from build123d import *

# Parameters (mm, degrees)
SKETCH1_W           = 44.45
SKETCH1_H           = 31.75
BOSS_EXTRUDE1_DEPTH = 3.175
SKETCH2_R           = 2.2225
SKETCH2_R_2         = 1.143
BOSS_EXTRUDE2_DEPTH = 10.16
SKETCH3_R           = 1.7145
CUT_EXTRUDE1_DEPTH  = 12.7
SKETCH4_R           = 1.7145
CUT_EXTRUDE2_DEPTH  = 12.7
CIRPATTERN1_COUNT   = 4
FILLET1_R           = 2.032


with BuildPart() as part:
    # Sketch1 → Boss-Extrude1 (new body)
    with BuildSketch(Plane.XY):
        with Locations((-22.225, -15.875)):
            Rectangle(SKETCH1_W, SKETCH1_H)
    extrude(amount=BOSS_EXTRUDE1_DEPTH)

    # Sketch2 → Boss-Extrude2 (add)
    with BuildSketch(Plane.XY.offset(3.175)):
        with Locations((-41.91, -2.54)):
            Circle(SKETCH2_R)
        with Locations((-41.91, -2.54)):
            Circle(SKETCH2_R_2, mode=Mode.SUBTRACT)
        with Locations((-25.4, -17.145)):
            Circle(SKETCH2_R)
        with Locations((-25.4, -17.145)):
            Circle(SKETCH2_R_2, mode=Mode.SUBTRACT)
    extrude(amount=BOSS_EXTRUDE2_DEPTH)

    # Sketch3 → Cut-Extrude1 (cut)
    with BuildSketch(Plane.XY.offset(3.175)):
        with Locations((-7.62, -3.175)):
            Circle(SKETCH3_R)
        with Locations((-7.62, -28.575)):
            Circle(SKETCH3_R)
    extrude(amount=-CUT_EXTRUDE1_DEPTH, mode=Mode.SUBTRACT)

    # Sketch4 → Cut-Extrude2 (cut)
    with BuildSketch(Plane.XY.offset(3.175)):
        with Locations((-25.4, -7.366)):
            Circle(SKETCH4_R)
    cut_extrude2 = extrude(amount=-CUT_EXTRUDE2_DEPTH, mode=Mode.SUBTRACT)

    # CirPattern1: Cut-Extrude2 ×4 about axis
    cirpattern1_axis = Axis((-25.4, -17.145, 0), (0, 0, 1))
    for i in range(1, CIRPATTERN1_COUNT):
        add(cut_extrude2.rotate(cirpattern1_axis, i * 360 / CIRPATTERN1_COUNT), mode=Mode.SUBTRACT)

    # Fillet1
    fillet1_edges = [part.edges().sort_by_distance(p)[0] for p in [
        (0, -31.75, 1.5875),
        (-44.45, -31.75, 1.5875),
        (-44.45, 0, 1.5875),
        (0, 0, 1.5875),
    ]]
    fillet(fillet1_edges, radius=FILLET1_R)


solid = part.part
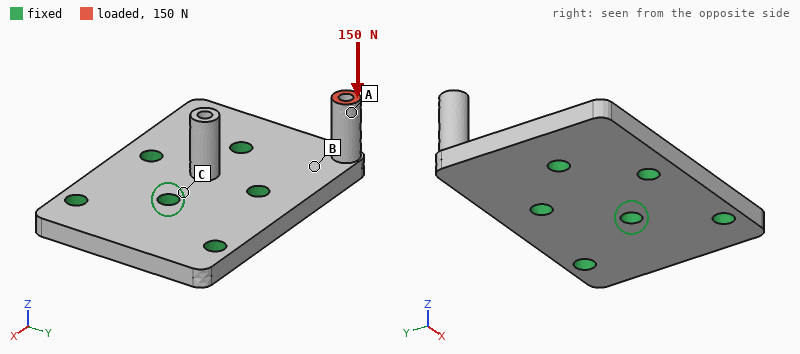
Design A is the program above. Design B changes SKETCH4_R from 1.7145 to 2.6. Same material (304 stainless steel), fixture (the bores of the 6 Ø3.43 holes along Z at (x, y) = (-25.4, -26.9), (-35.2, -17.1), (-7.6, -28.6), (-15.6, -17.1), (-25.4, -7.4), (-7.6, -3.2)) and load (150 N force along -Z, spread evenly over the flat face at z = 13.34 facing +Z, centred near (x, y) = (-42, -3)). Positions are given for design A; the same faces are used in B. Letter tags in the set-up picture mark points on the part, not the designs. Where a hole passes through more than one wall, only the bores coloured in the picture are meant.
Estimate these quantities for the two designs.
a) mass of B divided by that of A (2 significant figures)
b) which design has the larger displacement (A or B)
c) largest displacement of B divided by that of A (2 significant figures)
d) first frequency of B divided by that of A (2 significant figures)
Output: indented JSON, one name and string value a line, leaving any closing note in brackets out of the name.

{
  "mass of B divided by that of A": "0.97",
  "which design has the larger displacement": "A",
  "largest displacement of B divided by that of A": "0.88",
  "first frequency of B divided by that of A": "1.1"
}
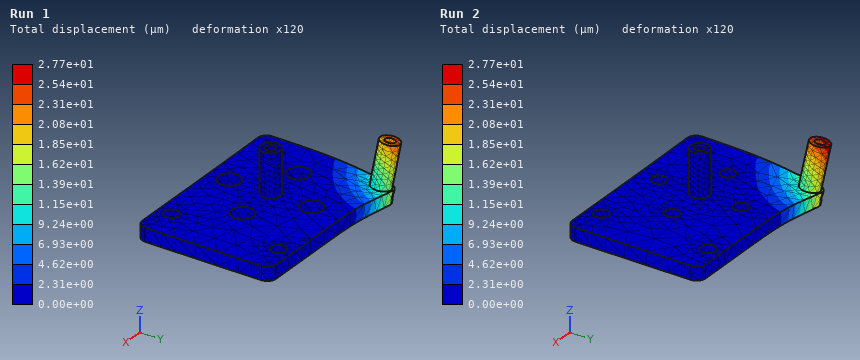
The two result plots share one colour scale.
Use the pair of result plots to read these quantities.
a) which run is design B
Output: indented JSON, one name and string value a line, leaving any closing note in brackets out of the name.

{
  "which run is design B": "Run 1"
}
